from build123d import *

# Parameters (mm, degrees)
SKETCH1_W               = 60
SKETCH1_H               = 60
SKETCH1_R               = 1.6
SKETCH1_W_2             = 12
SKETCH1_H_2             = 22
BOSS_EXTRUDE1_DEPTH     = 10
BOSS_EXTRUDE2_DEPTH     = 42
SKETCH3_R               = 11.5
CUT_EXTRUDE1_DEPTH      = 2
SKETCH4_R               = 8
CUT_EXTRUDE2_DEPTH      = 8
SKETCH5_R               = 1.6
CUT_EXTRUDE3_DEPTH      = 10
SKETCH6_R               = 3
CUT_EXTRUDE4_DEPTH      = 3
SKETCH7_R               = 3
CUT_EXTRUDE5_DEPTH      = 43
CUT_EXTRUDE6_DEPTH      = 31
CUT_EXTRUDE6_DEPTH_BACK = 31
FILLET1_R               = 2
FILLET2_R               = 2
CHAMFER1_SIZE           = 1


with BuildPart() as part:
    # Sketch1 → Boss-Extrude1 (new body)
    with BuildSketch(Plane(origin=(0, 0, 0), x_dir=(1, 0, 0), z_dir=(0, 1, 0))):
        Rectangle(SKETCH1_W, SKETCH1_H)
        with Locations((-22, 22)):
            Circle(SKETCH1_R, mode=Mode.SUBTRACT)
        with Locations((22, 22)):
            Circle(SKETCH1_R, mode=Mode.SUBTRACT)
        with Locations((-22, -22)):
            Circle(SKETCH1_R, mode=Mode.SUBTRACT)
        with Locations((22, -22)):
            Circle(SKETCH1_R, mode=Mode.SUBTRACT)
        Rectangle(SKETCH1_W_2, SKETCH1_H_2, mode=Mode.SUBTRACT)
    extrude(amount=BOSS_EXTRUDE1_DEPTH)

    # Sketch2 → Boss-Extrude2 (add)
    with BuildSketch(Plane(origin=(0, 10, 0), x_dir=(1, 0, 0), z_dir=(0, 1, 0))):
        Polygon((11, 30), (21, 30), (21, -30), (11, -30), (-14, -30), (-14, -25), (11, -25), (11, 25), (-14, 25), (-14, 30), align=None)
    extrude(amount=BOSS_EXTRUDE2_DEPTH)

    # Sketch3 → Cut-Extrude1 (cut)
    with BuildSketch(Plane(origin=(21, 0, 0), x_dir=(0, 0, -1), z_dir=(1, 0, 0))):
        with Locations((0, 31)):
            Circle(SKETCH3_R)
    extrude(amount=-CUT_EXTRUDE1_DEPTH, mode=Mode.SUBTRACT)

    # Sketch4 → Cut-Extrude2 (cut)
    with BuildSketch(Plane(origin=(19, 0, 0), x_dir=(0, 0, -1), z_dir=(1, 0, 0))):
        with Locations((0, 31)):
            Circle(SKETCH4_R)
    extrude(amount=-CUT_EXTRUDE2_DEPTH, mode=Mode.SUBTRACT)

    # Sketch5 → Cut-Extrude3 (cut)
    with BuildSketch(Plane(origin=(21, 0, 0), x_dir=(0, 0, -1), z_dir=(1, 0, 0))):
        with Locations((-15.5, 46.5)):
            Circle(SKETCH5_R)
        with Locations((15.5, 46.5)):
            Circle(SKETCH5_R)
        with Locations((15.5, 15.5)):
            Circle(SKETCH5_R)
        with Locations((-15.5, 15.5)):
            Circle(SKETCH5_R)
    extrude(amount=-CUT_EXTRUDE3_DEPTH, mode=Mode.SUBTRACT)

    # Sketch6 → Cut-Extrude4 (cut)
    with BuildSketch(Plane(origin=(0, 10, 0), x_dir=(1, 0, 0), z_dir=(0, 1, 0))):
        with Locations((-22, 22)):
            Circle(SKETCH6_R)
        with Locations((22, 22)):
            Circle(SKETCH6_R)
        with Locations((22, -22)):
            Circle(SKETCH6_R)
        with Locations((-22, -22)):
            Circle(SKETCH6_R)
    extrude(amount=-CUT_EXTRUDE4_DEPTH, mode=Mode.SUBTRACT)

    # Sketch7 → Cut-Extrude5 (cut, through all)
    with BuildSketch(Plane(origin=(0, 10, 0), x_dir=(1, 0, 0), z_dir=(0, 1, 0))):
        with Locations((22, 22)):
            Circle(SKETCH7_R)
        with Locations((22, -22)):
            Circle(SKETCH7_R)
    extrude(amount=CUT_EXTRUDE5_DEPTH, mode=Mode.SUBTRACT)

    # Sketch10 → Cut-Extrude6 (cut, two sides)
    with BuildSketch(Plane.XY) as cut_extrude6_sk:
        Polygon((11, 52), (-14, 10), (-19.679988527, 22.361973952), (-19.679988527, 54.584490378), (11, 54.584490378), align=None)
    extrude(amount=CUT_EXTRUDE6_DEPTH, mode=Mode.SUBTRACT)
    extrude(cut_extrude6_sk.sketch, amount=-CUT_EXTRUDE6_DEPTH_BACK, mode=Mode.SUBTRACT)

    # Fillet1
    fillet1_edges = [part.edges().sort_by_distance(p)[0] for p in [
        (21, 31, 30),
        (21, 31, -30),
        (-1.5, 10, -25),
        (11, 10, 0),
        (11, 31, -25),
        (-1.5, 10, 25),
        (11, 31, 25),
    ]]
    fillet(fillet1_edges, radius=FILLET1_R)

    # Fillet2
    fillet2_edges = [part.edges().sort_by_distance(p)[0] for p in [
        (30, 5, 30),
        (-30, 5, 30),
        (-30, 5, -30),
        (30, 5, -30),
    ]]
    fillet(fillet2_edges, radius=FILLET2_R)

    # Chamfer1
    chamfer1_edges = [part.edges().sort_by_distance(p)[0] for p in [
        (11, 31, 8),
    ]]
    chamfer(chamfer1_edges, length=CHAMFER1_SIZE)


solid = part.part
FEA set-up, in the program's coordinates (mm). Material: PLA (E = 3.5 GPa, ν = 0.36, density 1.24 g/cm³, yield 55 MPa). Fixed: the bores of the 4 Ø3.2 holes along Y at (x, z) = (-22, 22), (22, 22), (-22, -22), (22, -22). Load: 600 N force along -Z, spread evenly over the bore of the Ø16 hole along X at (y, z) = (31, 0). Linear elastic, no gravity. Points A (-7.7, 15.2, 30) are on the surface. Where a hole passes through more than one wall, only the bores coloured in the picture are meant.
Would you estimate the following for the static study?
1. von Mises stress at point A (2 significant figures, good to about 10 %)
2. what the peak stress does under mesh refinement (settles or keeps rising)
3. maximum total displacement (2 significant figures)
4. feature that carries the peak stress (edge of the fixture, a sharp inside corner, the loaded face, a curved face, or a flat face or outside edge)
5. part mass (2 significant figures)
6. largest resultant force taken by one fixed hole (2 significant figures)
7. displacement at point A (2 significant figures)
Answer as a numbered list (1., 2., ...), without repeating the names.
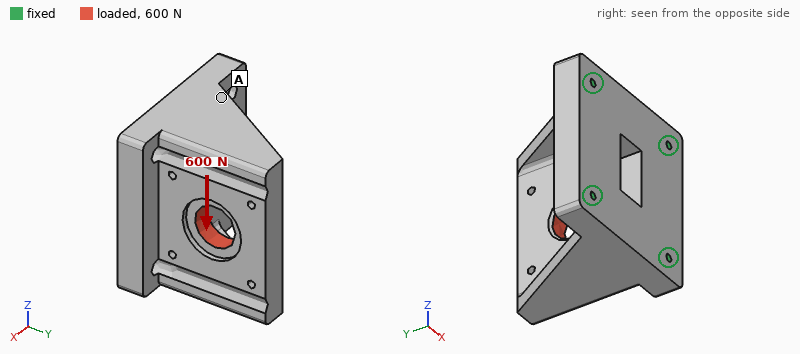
1. 1.4 MPa
2. keeps rising
3. 89 µm
4. edge of the fixture
5. 74 g
6. 410 N
7. 23 µm
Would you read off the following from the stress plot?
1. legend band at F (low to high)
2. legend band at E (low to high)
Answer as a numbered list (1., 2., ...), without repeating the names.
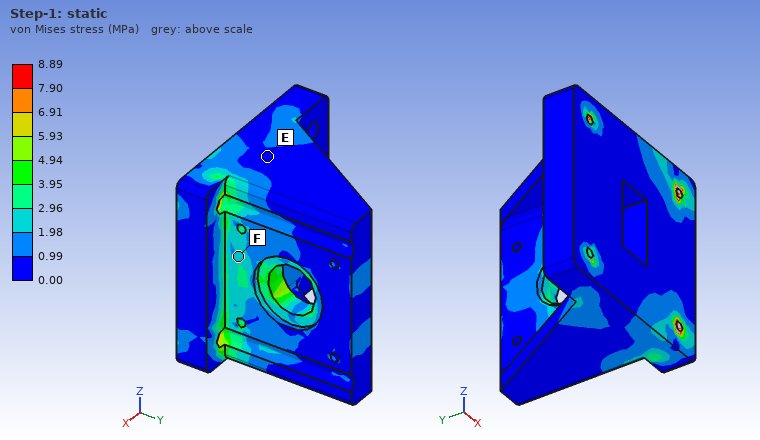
1. 1.98 to 2.96 MPa
2. 0.00 to 0.99 MPa
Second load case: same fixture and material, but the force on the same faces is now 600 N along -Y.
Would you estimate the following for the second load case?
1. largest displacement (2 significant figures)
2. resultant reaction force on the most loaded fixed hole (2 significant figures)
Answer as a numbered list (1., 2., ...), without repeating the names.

1. 34 µm
2. 270 N
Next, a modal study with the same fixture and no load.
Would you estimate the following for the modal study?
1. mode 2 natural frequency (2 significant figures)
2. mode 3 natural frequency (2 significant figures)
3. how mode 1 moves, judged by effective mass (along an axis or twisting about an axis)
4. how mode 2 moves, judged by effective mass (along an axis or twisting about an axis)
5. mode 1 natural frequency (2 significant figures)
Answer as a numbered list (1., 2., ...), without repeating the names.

1. 2600 Hz
2. 3100 Hz
3. along X
4. along Z
5. 1900 Hz
